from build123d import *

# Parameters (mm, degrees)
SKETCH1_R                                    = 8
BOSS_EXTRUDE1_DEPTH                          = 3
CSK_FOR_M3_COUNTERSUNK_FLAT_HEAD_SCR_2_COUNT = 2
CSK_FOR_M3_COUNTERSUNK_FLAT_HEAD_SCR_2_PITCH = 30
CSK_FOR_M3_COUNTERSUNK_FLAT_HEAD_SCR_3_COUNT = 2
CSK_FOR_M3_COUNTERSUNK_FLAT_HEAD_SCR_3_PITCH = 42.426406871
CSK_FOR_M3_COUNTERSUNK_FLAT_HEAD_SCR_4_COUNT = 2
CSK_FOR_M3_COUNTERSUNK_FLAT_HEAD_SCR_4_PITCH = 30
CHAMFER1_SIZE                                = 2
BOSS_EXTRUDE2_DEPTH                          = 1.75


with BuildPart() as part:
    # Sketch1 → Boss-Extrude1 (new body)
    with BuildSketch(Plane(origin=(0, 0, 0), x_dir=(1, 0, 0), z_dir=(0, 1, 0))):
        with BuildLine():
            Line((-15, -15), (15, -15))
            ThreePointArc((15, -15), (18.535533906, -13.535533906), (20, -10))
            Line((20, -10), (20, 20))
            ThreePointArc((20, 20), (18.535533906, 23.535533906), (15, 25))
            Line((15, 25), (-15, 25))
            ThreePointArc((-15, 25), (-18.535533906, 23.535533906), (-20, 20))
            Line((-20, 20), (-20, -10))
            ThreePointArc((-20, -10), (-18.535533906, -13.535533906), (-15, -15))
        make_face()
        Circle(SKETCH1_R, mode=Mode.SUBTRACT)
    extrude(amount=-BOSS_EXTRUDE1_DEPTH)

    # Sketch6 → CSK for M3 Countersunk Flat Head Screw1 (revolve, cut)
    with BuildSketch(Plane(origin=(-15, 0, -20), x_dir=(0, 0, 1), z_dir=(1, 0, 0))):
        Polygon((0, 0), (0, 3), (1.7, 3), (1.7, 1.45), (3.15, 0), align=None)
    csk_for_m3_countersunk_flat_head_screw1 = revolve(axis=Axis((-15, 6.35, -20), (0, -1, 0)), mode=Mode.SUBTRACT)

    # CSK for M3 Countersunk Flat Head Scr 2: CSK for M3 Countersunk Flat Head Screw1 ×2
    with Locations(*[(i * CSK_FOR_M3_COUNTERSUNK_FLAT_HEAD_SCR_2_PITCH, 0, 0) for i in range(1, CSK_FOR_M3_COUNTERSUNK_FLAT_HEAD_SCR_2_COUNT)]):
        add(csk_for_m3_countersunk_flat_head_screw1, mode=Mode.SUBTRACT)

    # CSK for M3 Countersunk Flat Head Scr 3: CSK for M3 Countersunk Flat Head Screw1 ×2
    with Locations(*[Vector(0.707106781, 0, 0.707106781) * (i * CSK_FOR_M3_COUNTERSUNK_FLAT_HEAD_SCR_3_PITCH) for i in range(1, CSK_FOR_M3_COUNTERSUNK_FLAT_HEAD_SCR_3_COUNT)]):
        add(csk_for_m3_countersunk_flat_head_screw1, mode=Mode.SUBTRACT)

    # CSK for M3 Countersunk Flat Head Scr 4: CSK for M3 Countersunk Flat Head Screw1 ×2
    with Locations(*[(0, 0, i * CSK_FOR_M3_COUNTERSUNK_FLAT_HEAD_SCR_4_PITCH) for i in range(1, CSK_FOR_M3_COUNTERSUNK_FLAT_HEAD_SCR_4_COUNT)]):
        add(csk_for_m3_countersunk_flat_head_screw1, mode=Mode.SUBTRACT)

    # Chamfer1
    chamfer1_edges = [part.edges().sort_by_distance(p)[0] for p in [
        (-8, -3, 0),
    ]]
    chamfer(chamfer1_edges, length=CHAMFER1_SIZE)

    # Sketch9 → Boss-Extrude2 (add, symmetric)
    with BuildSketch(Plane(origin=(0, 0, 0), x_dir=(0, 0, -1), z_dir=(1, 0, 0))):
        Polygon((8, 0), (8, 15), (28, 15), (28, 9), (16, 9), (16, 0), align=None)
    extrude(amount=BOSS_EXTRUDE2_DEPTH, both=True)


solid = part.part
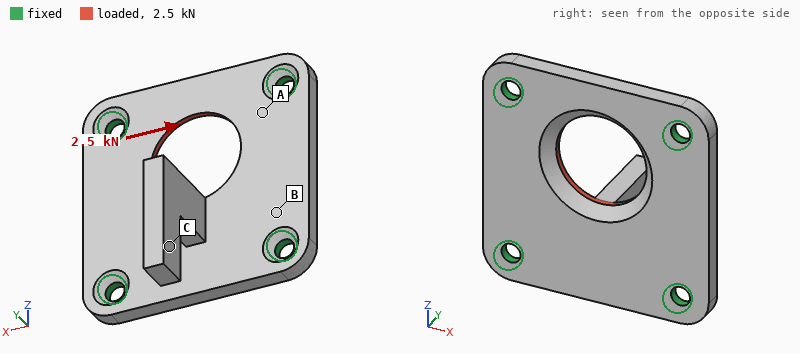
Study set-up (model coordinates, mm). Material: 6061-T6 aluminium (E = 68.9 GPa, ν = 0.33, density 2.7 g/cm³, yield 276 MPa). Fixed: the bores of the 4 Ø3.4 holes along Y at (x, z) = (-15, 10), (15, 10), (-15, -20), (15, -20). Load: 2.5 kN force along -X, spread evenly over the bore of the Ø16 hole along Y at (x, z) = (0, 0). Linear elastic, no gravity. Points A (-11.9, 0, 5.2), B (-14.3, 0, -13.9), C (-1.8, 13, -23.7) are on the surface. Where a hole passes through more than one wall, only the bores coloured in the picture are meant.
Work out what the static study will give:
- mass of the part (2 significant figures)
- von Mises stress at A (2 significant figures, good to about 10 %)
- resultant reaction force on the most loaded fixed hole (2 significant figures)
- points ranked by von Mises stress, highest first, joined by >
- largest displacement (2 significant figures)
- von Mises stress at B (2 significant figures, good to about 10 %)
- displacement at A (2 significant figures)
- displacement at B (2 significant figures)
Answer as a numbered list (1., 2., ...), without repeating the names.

1. 12 g
2. 34 MPa
3. 750 N
4. A > B > C
5. 13 µm
6. 19 MPa
7. 5.3 µm
8. 3.9 µm
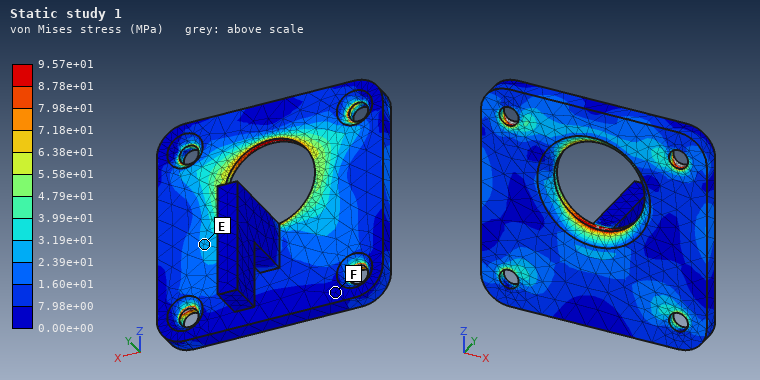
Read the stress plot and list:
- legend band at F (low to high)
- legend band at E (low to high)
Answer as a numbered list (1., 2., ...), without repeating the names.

1. 0.00e+00 to 7.98e+00 MPa
2. 2.39e+01 to 3.19e+01 MPa
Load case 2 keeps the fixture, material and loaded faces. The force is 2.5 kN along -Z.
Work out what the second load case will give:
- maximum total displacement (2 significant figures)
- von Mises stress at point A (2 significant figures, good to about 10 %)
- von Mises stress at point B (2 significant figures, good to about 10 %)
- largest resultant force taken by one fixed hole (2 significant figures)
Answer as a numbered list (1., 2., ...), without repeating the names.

1. 19 µm
2. 23 MPa
3. 16 MPa
4. 680 N
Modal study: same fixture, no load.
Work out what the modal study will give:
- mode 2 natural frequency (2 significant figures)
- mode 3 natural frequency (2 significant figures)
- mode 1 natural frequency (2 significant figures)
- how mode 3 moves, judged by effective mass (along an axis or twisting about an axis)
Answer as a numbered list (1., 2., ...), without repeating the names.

1. 6000 Hz
2. 8800 Hz
3. 5100 Hz
4. along Y
